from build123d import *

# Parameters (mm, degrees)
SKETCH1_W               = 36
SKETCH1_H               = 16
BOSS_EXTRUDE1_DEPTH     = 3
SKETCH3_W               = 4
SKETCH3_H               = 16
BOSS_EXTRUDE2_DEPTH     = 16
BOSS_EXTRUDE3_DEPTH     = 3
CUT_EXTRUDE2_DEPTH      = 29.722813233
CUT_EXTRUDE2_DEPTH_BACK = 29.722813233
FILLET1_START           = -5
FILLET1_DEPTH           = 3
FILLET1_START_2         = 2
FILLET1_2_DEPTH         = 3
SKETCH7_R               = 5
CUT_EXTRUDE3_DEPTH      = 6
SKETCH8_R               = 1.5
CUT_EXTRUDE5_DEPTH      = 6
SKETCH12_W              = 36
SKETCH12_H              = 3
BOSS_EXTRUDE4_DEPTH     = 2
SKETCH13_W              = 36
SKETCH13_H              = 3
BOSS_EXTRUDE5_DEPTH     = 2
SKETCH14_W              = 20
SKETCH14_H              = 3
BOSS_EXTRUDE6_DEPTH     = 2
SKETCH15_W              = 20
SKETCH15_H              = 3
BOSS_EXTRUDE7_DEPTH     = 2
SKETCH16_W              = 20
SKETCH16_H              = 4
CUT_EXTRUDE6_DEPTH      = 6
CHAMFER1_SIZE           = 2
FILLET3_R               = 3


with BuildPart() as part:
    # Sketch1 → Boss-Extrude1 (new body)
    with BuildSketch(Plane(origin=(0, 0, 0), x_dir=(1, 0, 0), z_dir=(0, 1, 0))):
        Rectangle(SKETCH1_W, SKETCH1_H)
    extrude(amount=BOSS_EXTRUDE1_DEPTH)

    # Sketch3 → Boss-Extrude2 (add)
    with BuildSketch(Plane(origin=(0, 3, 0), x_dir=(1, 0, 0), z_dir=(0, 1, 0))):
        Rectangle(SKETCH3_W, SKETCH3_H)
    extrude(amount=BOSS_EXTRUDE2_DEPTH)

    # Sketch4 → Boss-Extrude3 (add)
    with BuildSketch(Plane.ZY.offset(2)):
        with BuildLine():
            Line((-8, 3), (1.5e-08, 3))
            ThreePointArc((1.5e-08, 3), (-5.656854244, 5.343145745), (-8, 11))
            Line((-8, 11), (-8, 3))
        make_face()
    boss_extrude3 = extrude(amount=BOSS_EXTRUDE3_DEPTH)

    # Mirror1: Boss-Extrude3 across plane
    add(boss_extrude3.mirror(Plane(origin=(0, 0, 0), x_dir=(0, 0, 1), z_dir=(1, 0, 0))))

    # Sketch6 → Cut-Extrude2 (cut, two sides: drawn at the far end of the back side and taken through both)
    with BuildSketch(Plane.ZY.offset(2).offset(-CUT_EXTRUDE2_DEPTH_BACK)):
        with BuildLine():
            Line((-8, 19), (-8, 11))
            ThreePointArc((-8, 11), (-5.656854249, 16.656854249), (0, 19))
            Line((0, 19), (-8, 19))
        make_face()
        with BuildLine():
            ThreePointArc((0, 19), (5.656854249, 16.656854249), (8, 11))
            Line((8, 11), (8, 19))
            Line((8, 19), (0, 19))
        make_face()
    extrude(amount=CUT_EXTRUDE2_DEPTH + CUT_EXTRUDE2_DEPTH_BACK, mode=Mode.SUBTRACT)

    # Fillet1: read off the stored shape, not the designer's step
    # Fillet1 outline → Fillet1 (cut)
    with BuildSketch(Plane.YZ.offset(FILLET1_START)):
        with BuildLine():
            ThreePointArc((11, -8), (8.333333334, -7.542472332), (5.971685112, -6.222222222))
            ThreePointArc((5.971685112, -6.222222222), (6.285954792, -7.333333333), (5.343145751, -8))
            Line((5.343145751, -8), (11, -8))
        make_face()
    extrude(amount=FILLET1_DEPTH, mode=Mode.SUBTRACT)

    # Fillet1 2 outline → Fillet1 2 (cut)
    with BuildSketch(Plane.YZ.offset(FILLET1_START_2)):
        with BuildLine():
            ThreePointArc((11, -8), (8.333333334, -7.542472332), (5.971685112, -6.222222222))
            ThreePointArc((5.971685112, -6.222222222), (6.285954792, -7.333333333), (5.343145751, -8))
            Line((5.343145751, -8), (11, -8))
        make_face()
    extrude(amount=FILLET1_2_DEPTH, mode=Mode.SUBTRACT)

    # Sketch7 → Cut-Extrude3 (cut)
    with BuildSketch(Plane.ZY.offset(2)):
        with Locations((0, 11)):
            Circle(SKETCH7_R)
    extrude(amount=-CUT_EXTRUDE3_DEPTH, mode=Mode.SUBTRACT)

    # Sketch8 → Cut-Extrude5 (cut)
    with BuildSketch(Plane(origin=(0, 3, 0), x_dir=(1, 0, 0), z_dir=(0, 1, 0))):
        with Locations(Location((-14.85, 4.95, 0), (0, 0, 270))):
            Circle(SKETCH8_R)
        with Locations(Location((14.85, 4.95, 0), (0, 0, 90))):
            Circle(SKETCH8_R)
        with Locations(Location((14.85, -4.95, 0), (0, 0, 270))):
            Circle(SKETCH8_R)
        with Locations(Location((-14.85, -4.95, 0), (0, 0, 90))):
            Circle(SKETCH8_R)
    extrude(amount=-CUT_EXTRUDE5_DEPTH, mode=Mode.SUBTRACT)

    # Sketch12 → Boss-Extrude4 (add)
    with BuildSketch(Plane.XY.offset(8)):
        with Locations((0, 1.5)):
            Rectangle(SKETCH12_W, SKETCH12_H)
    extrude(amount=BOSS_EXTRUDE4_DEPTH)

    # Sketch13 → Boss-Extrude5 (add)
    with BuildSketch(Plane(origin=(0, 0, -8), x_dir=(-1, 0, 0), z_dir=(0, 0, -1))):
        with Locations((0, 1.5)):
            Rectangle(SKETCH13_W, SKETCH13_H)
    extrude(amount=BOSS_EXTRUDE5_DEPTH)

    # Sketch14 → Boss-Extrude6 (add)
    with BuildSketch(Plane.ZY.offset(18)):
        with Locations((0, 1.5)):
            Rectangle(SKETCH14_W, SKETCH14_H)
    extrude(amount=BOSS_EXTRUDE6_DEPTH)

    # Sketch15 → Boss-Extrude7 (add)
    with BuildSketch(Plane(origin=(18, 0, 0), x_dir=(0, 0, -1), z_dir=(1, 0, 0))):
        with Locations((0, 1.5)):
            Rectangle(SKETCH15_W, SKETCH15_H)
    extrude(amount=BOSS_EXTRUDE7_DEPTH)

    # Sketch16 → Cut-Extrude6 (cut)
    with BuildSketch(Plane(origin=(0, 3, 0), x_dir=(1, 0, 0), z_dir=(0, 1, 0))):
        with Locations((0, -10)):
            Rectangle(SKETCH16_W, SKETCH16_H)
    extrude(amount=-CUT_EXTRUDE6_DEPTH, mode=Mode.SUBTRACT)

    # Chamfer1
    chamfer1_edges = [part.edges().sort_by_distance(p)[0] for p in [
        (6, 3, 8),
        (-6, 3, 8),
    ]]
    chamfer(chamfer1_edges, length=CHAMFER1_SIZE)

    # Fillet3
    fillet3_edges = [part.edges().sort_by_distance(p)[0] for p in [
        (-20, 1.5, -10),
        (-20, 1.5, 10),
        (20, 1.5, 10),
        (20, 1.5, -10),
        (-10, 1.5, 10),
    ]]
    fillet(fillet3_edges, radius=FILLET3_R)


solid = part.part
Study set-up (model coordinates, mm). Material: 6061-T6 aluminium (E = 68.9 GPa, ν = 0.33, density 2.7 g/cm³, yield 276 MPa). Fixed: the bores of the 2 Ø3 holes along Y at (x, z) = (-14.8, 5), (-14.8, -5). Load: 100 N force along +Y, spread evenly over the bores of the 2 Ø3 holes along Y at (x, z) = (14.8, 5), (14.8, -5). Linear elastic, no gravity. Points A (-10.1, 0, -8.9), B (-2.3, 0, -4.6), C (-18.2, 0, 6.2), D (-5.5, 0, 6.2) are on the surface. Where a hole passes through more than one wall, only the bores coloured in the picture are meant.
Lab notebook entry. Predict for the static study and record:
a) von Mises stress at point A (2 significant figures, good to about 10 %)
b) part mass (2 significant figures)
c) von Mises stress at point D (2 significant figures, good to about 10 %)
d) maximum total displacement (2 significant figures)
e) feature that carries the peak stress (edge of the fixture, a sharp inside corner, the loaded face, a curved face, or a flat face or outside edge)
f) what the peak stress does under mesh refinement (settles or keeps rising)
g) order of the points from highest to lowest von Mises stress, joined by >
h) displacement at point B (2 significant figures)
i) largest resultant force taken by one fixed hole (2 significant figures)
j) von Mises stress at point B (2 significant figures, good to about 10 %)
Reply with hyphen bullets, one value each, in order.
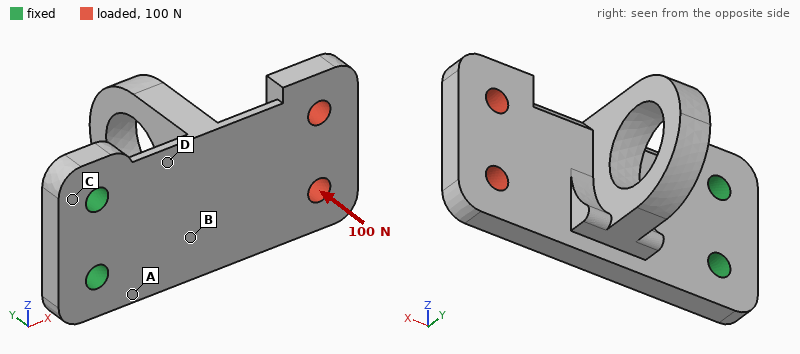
- 92 MPa
- 7.6 g
- 70 MPa
- 0.33 mm
- edge of the fixture
- keeps rising
- A > D > B > C
- 0.066 mm
- 54 N
- 42 MPa
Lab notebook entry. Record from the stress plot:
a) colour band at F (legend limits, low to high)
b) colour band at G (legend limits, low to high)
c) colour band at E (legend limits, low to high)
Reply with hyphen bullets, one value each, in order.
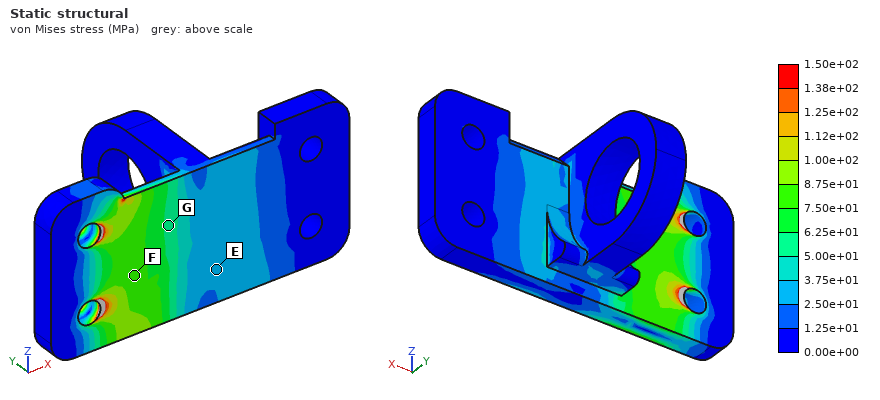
- 7.50e+01 to 8.75e+01 MPa
- 5.00e+01 to 6.25e+01 MPa
- 2.50e+01 to 3.75e+01 MPa
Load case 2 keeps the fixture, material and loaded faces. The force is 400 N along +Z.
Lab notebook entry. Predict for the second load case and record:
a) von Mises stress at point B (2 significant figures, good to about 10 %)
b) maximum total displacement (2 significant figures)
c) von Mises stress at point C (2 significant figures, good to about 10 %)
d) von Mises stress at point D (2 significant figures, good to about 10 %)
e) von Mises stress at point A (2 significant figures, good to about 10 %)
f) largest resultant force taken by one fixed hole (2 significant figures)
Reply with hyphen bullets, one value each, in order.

- 29 MPa
- 65 µm
- 10.0 MPa
- 43 MPa
- 45 MPa
- 1.0 kN
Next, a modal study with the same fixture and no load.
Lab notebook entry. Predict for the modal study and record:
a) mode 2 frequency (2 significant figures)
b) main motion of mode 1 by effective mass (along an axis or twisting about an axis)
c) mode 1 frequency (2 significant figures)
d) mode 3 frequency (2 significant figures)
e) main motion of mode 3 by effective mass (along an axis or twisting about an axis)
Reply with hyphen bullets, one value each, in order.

- 6200 Hz
- along Y
- 2000 Hz
- 9200 Hz
- along Z
